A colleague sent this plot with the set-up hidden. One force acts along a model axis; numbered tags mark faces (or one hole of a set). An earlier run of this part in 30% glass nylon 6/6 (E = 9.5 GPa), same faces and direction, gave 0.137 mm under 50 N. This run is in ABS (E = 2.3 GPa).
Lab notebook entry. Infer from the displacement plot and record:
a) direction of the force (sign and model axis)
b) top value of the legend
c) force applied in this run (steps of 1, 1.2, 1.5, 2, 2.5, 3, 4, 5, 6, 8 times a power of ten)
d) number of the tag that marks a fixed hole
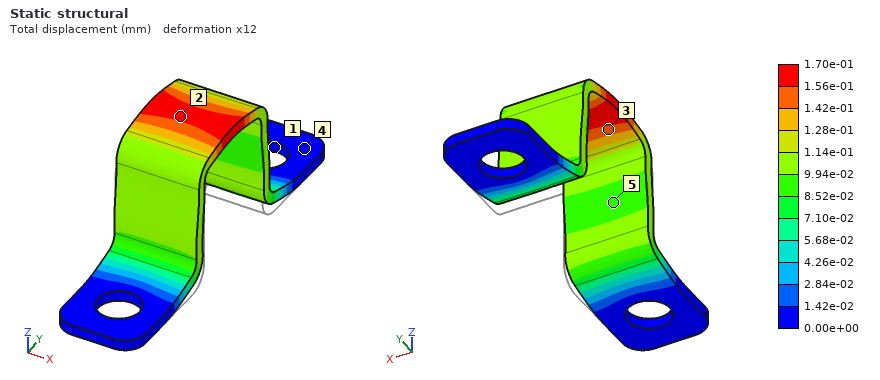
+Z
1.70e-01 mm
15 N
1
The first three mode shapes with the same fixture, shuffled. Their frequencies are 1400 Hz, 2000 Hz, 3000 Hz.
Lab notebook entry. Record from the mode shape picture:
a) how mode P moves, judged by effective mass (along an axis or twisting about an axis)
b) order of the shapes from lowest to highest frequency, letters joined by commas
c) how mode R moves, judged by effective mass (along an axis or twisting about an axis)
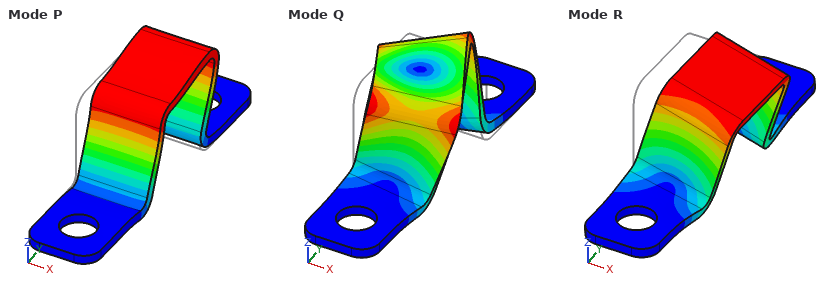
along Y
R, P, Q
along X
